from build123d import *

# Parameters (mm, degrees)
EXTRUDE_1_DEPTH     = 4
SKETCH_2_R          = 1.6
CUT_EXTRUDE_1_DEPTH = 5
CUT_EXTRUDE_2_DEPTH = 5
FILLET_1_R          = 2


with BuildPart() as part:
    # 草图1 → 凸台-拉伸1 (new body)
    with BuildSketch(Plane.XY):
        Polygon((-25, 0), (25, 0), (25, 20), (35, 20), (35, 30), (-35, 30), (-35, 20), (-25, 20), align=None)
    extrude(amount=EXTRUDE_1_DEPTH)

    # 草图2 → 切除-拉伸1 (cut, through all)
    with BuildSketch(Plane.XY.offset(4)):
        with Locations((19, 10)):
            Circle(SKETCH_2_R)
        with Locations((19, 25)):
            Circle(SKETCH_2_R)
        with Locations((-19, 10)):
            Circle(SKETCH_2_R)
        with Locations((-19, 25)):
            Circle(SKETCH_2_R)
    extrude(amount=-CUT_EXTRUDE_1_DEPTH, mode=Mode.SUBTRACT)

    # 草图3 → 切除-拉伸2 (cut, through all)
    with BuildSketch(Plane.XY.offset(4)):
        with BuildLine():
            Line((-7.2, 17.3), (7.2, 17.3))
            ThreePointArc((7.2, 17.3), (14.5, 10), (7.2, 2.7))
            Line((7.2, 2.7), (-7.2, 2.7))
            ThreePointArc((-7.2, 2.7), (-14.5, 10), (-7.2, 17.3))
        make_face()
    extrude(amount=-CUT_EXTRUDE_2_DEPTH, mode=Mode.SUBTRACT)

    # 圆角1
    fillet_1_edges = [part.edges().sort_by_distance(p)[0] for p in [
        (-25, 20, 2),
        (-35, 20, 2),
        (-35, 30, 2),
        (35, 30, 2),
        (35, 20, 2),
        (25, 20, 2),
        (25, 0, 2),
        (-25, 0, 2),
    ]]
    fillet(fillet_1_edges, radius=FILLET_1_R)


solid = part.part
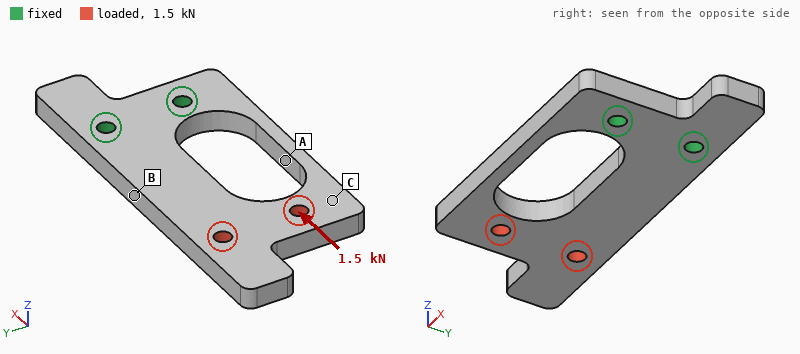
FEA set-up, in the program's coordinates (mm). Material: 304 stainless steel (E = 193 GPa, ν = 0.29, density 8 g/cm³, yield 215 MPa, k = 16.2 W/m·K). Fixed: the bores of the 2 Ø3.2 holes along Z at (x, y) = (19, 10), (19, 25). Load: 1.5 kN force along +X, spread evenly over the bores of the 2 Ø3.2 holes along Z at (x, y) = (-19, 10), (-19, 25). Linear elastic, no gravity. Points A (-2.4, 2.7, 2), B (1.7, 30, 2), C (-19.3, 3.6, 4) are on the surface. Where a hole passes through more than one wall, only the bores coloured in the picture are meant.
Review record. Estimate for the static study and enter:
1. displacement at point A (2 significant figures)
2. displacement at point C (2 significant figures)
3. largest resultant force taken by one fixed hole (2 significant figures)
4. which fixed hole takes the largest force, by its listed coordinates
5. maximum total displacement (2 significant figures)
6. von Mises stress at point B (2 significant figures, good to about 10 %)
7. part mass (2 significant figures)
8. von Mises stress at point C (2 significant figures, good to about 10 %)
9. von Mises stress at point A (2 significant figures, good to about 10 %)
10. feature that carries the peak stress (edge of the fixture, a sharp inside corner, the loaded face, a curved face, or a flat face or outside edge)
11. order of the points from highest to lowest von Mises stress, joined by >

10 µm
10 µm
840 N
(19, 25)
12 µm
7.4 MPa
41 g
19 MPa
46 MPa
edge of the fixture
A > C > B
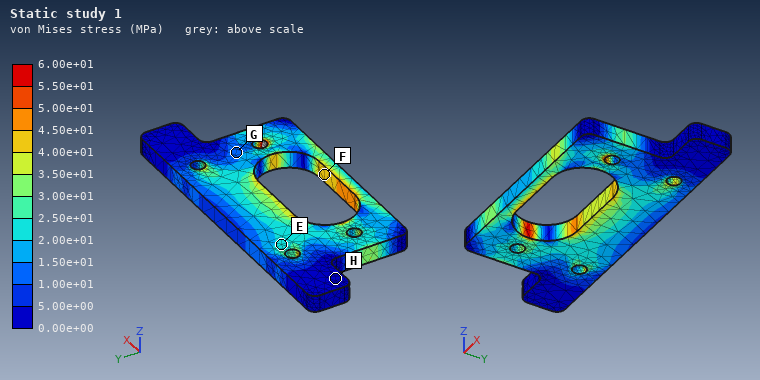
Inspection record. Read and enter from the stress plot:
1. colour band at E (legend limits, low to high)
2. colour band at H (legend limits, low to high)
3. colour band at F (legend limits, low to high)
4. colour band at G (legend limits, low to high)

2.00e+01 to 2.50e+01 MPa
0.00e+00 to 5.00e+00 MPa
4.00e+01 to 4.50e+01 MPa
1.00e+01 to 1.50e+01 MPa
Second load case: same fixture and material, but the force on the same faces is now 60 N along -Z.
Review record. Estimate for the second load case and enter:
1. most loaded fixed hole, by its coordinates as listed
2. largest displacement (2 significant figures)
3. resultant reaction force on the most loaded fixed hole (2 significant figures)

(19, 25)
99 µm
44 N
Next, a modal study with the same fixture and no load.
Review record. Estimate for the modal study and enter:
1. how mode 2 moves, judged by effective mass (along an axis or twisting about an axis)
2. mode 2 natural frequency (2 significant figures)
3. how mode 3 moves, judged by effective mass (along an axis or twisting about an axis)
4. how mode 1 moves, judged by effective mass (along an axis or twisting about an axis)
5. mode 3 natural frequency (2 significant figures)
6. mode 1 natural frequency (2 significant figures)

twisting about X
3600 Hz
along Y
along Z
4700 Hz
1100 Hz
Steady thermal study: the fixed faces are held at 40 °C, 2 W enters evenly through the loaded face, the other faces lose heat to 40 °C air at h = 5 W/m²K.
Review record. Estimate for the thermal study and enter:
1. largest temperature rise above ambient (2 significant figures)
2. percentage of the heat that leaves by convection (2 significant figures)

58 K
25 %
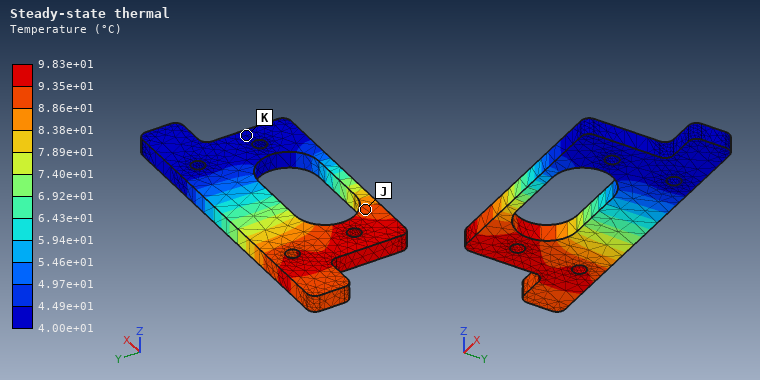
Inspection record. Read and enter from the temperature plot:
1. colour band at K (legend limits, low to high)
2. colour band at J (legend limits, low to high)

4.00e+01 to 4.49e+01 °C
8.86e+01 to 9.35e+01 °C
